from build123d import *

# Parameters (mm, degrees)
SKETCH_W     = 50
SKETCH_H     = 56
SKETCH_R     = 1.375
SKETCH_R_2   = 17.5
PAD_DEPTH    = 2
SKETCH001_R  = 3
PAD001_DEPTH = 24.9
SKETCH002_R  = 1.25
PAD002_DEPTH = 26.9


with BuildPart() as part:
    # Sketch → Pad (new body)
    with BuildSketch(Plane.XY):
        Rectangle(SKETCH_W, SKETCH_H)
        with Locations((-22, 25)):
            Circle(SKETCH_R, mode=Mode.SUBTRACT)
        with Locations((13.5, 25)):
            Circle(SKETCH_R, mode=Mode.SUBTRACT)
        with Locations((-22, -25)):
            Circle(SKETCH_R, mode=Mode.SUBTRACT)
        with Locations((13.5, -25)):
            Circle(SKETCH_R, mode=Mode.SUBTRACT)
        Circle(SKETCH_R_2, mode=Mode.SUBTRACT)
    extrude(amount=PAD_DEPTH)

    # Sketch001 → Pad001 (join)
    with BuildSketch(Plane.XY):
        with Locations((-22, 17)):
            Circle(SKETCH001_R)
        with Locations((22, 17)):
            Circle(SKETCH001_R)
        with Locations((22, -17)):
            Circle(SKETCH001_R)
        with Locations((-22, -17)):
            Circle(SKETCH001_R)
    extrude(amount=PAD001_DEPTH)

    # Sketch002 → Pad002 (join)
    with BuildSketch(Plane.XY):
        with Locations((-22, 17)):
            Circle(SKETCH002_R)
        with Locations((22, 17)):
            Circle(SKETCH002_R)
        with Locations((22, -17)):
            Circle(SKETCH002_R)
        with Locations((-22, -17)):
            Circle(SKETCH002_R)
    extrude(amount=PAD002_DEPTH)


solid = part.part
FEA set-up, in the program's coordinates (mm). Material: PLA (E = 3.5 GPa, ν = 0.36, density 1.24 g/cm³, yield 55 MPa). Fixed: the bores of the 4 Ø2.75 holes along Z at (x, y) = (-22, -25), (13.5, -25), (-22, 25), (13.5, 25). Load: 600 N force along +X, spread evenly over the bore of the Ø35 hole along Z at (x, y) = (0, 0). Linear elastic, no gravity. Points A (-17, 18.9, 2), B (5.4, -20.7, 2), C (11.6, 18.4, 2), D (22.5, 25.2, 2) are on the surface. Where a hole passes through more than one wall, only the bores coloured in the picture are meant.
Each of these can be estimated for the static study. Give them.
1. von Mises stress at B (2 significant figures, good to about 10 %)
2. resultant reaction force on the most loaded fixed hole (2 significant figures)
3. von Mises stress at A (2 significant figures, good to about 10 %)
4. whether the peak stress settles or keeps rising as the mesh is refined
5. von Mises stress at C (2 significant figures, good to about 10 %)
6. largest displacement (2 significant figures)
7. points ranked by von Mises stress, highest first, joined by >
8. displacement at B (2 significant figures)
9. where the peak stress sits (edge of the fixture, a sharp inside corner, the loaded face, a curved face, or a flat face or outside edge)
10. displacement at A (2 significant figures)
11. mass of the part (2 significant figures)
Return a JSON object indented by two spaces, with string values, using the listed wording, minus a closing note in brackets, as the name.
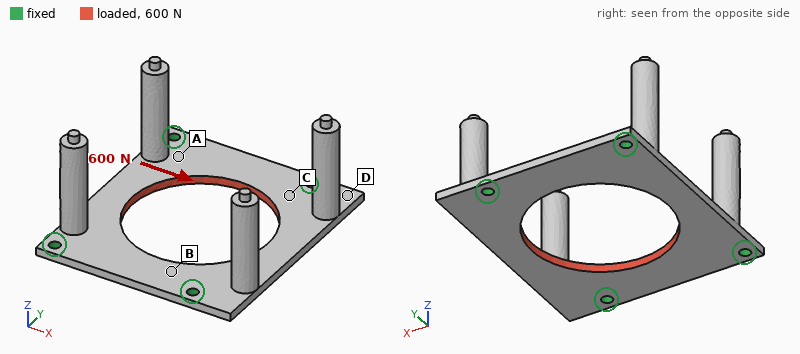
{
  "von Mises stress at B": "8.4 MPa",
  "resultant reaction force on the most loaded fixed hole": "180 N",
  "von Mises stress at A": "3.8 MPa",
  "whether the peak stress settles or keeps rising as the mesh is refined": "keeps rising",
  "von Mises stress at C": "5.9 MPa",
  "largest displacement": "0.13 mm",
  "points ranked by von Mises stress, highest first, joined by >": "B > C > A > D",
  "displacement at B": "0.029 mm",
  "where the peak stress sits": "edge of the fixture",
  "displacement at A": "0.034 mm",
  "mass of the part": "7.8 g"
}
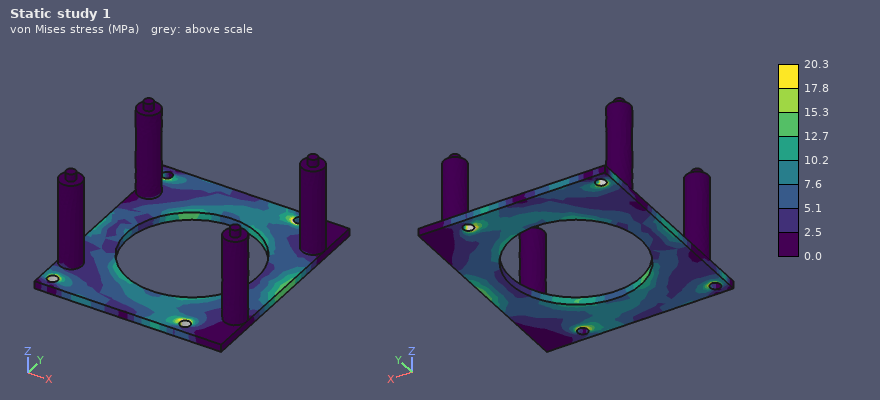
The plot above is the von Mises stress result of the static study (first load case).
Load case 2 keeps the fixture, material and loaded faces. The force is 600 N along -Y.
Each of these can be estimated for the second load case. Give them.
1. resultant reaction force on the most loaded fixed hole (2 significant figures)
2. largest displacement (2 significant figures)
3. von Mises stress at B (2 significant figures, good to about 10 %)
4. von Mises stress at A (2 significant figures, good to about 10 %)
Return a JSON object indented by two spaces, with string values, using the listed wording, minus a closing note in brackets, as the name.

{
  "resultant reaction force on the most loaded fixed hole": "170 N",
  "largest displacement": "59 µm",
  "von Mises stress at B": "5.9 MPa",
  "von Mises stress at A": "4.2 MPa"
}
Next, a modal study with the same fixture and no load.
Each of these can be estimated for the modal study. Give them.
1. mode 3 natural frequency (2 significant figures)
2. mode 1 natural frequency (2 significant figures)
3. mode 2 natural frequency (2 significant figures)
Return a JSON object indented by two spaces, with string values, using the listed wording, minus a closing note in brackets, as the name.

{
  "mode 3 natural frequency": "830 Hz",
  "mode 1 natural frequency": "630 Hz",
  "mode 2 natural frequency": "770 Hz"
}
